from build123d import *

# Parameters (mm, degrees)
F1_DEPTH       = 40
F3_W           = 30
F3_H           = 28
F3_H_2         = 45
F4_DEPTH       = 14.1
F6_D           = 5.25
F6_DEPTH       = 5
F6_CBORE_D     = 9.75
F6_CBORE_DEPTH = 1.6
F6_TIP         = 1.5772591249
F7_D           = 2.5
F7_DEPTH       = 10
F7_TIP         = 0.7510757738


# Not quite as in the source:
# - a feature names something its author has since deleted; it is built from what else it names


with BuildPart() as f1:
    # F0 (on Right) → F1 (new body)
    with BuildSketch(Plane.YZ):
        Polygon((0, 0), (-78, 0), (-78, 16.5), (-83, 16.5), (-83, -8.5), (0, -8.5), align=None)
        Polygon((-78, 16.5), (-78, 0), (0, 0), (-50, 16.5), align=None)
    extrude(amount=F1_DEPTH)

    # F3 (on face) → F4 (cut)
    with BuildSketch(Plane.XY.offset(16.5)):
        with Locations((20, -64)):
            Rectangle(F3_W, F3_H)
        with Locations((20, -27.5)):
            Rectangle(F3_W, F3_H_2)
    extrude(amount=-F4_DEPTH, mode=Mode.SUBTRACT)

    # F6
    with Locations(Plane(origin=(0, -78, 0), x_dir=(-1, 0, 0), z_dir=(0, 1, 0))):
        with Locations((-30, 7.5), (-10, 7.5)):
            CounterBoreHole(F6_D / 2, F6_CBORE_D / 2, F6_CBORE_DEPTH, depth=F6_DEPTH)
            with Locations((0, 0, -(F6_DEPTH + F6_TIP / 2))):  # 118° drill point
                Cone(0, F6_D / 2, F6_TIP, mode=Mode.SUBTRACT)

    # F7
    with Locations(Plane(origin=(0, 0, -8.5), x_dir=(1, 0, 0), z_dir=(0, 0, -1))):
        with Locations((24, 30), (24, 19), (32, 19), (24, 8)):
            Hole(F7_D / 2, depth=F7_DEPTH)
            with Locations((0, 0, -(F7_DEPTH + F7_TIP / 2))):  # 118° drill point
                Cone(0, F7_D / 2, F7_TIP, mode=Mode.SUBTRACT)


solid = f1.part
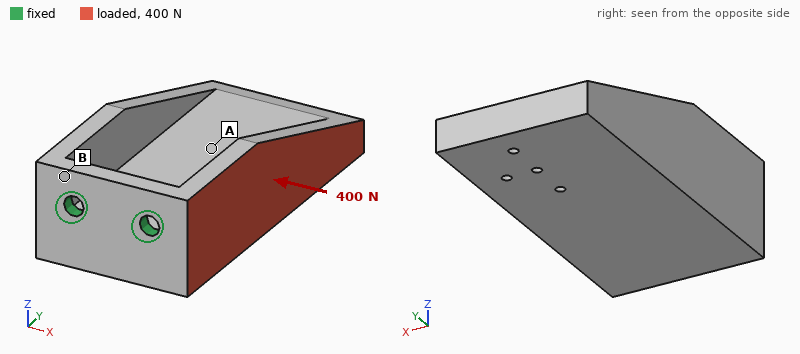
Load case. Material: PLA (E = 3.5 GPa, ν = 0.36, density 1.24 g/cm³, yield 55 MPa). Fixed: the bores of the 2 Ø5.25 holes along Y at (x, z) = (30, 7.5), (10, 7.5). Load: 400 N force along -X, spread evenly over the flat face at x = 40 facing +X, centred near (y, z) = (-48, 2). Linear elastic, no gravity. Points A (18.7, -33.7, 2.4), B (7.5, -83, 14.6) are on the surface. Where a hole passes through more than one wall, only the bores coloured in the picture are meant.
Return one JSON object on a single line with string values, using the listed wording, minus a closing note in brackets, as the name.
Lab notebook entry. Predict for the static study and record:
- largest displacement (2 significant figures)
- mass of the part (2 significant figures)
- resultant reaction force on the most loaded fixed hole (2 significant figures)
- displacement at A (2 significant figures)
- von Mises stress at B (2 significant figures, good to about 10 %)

{"largest displacement": "0.67 mm", "mass of the part": "56 g", "resultant reaction force on the most loaded fixed hole": "590 N", "displacement at A": "0.40 mm", "von Mises stress at B": "8.9 MPa"}
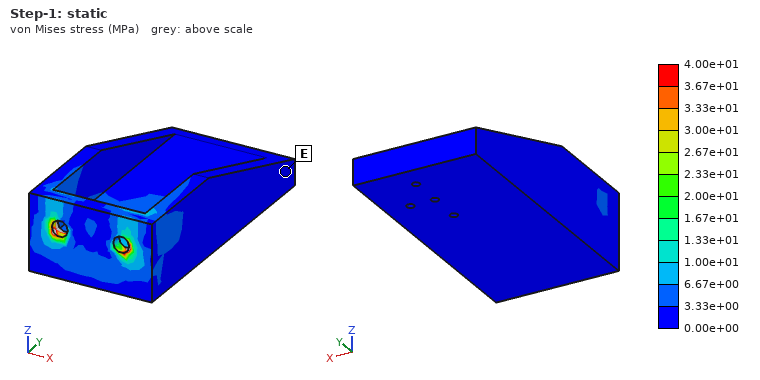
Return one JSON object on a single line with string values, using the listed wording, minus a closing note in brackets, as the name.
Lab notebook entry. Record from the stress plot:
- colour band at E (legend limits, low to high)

{"colour band at E": "0.00e+00 to 3.33e+00 MPa"}
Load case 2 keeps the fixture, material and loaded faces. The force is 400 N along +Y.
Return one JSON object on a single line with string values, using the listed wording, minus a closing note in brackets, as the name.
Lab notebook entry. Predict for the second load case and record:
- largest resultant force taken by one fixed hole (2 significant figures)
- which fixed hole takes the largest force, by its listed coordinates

{"largest resultant force taken by one fixed hole": "520 N", "which fixed hole takes the largest force, by its listed coordinates": "(30, 7.5)"}
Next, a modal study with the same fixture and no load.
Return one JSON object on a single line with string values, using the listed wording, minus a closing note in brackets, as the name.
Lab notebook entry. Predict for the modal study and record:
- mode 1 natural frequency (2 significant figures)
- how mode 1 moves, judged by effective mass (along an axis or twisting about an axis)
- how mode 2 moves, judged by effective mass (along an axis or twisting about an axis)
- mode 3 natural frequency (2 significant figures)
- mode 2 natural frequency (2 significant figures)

{"mode 1 natural frequency": "260 Hz", "how mode 1 moves, judged by effective mass": "along Z", "how mode 2 moves, judged by effective mass": "along X", "mode 3 natural frequency": "1500 Hz", "mode 2 natural frequency": "640 Hz"}
